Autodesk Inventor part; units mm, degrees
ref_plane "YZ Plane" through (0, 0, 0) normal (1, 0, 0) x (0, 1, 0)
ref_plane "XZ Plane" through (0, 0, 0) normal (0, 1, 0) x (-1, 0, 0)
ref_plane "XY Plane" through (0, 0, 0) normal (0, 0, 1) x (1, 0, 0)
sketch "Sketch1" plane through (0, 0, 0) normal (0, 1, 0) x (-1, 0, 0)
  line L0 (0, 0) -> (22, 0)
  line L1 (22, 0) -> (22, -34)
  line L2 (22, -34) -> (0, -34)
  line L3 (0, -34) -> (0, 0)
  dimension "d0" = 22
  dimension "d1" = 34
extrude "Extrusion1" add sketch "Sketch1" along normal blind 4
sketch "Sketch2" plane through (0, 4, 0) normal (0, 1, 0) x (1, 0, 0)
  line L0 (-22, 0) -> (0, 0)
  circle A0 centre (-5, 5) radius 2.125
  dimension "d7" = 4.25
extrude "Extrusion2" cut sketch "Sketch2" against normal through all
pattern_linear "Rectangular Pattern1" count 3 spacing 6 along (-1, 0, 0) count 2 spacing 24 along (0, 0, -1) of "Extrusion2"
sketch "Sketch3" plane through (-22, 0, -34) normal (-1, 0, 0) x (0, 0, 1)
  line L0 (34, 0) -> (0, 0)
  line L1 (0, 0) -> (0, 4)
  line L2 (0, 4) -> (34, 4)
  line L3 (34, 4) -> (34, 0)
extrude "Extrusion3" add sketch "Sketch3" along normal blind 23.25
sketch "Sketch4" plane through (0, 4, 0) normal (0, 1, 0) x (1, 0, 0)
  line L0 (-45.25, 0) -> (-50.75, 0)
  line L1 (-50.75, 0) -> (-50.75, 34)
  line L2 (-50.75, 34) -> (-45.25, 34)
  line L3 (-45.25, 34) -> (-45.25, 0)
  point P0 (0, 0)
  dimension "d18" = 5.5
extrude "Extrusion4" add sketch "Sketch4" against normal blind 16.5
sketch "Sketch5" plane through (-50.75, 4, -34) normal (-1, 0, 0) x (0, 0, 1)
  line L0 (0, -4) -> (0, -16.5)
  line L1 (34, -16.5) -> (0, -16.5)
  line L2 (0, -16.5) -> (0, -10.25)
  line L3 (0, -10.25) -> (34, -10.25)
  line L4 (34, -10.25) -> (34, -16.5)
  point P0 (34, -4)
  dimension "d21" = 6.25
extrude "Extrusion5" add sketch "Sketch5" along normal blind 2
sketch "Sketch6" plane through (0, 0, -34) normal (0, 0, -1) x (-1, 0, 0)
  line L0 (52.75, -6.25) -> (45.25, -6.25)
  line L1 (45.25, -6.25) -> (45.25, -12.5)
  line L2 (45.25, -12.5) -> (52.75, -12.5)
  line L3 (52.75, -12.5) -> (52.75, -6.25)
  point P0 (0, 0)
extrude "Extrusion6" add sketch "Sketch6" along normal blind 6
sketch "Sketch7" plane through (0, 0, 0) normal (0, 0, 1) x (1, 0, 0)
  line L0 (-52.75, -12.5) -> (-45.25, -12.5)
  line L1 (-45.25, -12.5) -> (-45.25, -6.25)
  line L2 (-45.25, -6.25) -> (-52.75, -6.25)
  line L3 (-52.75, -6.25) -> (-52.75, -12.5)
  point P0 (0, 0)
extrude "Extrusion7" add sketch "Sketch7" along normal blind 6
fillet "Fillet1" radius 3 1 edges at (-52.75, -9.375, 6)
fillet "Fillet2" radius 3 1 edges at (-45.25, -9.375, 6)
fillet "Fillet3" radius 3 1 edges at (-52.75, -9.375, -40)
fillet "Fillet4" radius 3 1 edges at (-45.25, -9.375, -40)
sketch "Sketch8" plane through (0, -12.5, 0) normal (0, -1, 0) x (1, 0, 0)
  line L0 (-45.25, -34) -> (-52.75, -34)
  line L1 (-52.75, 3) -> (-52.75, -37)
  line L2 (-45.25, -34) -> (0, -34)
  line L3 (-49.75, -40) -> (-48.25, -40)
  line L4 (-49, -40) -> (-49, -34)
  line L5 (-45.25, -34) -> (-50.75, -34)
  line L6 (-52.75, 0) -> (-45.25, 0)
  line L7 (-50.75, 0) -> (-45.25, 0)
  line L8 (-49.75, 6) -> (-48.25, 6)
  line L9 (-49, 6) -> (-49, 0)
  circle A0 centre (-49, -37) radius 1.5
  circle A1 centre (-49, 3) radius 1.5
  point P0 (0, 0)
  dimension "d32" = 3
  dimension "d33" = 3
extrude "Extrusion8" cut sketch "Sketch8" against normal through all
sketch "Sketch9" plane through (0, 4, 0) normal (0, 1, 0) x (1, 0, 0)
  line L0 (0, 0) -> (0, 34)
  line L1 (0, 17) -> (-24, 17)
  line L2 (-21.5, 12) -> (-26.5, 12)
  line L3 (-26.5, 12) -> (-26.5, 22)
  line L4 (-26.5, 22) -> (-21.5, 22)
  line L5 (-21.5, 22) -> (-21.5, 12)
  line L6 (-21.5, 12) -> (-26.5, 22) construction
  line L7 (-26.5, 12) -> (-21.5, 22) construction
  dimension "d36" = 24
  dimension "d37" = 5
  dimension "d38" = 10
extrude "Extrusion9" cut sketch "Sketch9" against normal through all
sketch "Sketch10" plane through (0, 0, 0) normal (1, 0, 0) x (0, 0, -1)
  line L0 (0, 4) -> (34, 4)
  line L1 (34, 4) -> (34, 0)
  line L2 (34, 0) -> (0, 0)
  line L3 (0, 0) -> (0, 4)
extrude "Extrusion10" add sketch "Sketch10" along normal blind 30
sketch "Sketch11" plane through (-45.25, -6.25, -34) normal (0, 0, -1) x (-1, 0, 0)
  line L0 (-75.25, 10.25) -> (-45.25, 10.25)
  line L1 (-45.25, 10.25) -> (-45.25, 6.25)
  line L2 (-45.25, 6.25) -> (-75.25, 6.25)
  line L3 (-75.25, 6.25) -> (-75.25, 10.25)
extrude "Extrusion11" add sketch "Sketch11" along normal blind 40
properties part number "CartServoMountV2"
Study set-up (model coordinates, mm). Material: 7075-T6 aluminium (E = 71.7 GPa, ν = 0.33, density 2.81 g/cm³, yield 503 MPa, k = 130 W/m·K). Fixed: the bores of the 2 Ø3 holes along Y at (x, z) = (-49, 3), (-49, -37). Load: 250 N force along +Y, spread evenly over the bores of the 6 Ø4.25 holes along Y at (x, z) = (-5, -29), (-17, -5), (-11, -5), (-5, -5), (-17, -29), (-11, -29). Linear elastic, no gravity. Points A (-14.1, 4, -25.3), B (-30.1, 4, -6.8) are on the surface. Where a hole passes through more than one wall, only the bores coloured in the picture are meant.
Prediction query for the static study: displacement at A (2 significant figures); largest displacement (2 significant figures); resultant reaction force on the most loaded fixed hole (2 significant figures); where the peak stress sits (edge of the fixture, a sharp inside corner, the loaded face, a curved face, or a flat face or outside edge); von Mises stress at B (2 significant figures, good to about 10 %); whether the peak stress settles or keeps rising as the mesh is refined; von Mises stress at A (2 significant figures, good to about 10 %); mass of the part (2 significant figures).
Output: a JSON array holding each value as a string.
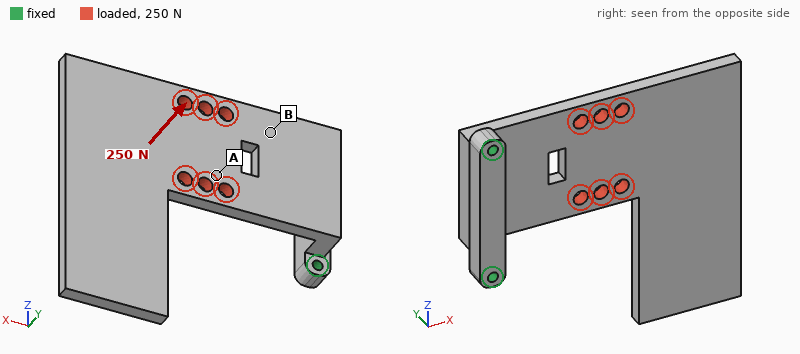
["0.46 mm", "1.3 mm", "180 N", "edge of the fixture", "58 MPa", "keeps rising", "15 MPa", "52 g"]
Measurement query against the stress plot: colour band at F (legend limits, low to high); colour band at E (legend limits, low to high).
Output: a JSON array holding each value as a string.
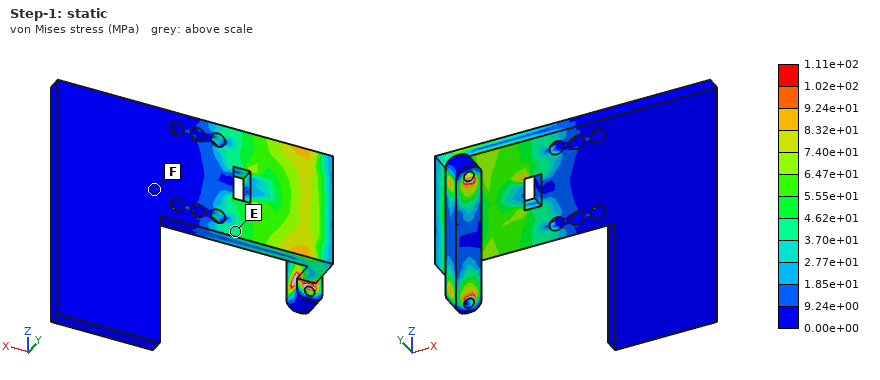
["0.00e+00 to 9.24e+00 MPa", "3.70e+01 to 4.62e+01 MPa"]
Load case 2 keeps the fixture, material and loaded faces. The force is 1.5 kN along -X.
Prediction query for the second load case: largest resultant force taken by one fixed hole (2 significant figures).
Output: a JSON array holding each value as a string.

["750 N"]
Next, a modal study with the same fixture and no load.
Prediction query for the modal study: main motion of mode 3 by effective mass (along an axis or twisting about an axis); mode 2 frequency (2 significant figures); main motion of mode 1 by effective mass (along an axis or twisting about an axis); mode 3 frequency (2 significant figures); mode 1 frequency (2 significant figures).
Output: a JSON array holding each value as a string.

["along Z", "770 Hz", "along Y", "1200 Hz", "290 Hz"]
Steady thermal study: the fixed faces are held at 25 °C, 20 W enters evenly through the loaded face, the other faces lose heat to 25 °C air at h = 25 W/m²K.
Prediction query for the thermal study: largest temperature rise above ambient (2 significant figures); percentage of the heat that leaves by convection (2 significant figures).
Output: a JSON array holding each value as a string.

["45 K", "37 %"]
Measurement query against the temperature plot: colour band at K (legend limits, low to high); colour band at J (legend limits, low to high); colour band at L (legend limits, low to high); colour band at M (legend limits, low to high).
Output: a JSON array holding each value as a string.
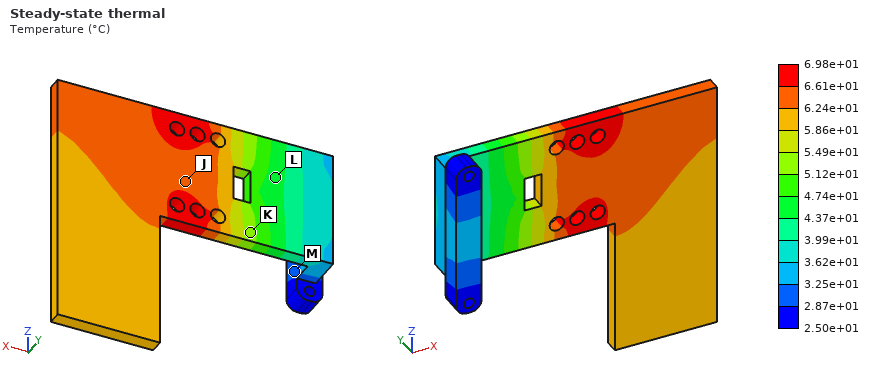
["5.12e+01 to 5.49e+01 °C", "6.24e+01 to 6.61e+01 °C", "4.37e+01 to 4.74e+01 °C", "2.87e+01 to 3.25e+01 °C"]
